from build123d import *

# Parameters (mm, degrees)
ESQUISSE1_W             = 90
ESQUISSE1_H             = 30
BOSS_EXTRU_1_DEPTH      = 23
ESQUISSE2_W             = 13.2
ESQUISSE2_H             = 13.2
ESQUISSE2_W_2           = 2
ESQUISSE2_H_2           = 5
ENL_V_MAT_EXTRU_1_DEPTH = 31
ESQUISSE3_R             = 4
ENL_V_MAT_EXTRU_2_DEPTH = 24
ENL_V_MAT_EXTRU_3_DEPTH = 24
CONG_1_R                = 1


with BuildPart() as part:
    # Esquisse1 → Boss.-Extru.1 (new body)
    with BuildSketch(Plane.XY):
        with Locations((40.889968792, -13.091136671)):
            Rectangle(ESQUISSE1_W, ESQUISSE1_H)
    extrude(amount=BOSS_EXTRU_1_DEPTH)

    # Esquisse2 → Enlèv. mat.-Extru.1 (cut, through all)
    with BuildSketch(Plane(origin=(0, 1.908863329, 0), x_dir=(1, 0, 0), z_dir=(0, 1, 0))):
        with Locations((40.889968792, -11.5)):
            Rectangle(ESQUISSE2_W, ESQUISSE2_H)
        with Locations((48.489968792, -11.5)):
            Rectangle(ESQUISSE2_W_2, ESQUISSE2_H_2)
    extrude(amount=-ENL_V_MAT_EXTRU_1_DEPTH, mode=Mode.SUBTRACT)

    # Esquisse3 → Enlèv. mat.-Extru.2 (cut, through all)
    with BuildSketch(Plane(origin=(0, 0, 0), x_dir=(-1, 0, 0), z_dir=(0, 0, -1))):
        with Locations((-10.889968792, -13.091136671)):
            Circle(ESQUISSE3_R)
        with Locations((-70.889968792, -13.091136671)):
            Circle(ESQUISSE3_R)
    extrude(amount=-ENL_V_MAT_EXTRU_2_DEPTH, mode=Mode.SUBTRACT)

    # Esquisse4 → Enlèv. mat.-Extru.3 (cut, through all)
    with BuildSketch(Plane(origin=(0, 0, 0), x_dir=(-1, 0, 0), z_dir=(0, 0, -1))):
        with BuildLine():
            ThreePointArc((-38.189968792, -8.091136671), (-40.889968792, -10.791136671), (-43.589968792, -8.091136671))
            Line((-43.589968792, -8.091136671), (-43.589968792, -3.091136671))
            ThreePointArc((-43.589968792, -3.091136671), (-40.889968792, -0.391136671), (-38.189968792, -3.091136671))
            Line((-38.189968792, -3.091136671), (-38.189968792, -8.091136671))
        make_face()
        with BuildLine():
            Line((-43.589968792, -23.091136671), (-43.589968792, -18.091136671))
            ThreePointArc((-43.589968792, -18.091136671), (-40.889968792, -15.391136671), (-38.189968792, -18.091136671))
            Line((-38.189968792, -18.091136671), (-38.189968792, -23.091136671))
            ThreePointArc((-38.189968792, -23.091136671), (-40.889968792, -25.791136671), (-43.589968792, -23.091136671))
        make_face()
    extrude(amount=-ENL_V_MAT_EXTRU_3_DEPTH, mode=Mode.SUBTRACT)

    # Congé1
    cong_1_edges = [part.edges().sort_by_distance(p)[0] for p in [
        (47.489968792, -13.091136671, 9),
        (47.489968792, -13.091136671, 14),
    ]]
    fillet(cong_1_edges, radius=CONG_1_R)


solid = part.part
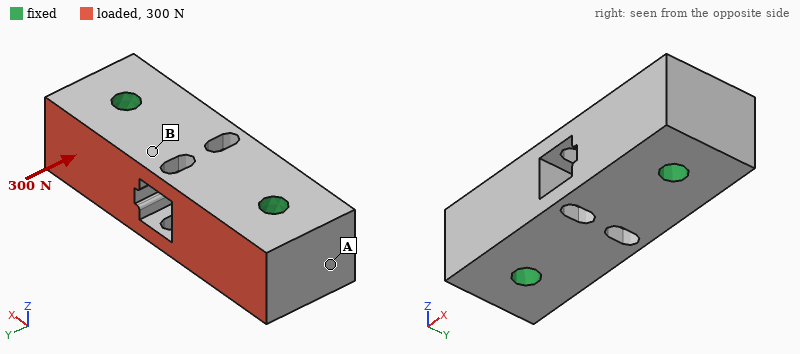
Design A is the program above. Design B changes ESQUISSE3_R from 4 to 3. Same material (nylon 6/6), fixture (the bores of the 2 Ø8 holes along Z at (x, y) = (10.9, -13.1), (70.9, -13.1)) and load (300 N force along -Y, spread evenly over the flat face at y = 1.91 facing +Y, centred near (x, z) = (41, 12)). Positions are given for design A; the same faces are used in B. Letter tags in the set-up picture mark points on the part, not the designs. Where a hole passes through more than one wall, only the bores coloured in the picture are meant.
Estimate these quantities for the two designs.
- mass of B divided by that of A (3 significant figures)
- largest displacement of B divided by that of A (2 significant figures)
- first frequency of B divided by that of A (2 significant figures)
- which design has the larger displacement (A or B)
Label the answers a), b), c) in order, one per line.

a) 1.02
b) 1.2
c) 0.84
d) B
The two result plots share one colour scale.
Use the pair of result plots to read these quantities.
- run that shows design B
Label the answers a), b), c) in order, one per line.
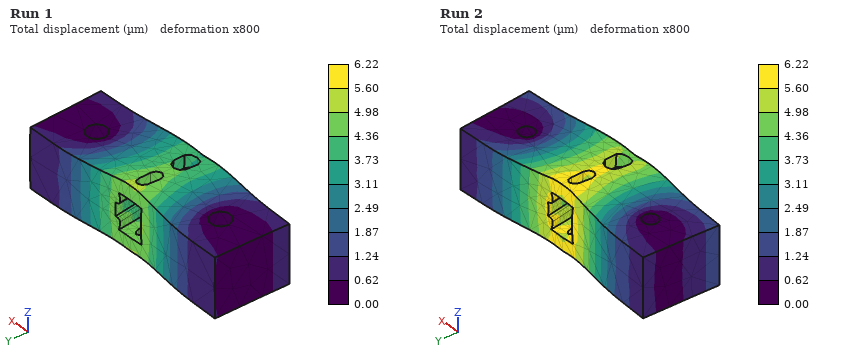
a) Run 2
